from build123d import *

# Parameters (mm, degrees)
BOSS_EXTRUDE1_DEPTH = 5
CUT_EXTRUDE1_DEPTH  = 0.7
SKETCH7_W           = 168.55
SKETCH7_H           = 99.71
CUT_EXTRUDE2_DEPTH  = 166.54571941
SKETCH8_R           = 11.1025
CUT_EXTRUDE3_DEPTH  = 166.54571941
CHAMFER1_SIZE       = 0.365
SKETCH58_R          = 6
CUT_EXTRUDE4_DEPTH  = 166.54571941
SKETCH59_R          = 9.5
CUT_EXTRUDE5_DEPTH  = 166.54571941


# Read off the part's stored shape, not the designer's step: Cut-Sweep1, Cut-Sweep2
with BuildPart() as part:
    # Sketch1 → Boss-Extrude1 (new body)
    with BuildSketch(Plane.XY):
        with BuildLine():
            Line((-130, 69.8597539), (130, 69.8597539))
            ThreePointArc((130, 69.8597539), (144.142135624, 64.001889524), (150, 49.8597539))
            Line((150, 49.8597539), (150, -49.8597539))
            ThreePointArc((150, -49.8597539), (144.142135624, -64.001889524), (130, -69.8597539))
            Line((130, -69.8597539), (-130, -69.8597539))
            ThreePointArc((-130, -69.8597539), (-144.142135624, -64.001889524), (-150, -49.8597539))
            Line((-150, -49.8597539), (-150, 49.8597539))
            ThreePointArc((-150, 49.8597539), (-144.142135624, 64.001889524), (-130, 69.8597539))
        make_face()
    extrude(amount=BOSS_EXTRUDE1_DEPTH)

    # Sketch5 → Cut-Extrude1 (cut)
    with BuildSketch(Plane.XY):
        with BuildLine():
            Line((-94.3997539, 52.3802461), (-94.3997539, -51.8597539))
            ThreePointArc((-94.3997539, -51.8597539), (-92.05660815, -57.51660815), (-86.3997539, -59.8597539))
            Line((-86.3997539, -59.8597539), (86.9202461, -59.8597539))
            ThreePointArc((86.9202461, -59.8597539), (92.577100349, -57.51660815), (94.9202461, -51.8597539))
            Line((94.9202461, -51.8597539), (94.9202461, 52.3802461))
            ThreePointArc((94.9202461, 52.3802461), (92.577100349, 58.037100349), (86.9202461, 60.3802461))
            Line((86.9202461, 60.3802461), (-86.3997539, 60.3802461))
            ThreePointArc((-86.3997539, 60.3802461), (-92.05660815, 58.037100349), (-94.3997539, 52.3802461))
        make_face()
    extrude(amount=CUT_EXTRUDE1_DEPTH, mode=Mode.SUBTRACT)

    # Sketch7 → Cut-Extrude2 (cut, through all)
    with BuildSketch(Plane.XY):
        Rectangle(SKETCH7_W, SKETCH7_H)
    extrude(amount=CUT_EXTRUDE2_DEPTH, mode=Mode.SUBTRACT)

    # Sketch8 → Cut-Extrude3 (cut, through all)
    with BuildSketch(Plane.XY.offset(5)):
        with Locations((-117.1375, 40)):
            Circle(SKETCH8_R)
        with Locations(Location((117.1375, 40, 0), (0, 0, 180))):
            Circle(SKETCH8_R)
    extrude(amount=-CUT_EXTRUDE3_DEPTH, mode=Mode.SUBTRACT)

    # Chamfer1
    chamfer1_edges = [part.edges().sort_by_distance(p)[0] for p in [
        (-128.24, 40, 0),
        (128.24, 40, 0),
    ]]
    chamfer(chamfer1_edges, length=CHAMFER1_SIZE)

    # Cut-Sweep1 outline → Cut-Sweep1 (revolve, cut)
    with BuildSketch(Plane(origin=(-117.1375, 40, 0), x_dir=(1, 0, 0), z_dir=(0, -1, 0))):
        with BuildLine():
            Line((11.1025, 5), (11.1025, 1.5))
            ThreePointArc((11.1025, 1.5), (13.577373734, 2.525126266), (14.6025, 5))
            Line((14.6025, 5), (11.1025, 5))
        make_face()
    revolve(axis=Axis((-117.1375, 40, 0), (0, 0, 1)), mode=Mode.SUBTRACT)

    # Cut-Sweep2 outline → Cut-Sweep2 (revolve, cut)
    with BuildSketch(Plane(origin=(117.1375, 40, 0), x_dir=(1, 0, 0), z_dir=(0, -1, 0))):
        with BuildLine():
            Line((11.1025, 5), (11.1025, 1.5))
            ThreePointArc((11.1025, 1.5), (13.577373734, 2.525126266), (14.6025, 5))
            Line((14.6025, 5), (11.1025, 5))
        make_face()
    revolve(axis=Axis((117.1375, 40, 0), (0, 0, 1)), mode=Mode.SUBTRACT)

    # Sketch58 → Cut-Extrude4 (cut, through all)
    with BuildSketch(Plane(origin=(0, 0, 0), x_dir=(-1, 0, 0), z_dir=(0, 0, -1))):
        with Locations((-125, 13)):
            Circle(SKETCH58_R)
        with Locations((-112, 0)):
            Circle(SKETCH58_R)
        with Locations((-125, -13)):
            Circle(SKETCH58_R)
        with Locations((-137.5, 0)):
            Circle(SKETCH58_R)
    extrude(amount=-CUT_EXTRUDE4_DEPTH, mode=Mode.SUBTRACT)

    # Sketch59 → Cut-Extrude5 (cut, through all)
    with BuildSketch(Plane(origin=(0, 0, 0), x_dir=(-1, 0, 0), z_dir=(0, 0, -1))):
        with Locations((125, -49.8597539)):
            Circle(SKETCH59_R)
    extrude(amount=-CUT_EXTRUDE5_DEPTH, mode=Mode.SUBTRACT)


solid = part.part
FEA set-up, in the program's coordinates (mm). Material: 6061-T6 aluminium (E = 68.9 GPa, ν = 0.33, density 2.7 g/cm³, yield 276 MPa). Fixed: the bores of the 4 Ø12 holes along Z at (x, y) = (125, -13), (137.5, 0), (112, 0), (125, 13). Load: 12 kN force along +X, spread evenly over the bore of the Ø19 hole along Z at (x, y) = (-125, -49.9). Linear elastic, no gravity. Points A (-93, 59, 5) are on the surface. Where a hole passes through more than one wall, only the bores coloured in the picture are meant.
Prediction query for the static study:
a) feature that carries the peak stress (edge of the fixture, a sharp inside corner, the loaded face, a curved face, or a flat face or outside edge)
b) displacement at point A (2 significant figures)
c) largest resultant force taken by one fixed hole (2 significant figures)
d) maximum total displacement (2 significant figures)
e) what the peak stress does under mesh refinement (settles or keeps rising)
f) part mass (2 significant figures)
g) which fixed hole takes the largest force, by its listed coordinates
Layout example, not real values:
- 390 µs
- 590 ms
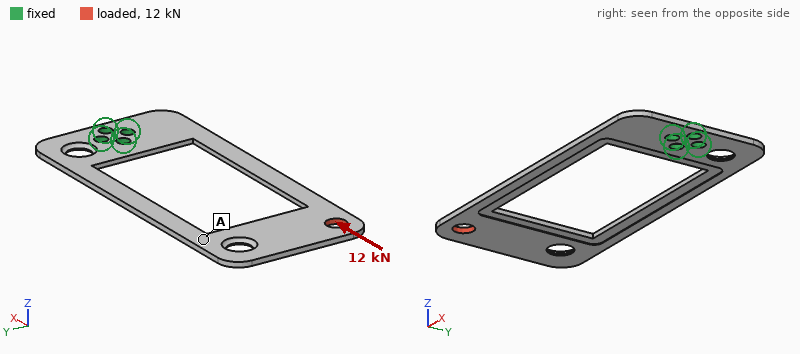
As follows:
- edge of the fixture
- 1.7 mm
- 14 kN
- 2.8 mm
- keeps rising
- 300 g
- (125, -13)
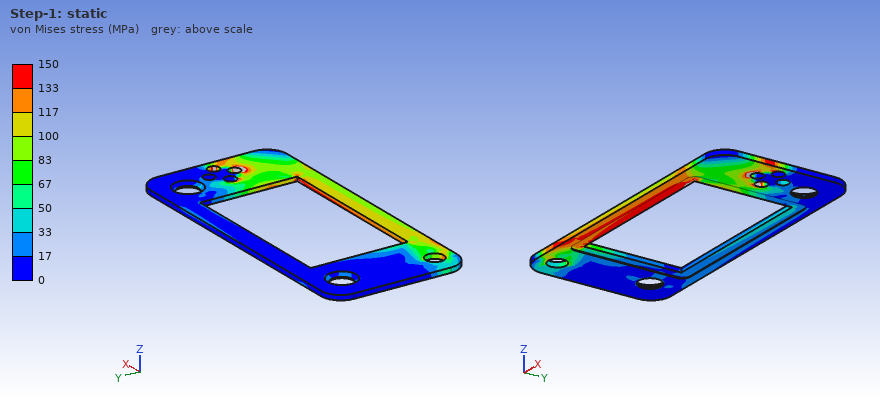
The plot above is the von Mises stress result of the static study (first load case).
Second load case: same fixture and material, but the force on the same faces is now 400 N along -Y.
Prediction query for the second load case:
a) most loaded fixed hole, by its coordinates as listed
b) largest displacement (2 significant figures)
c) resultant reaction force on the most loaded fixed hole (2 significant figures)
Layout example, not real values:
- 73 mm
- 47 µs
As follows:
- (112, 0)
- 0.74 mm
- 1.9 kN
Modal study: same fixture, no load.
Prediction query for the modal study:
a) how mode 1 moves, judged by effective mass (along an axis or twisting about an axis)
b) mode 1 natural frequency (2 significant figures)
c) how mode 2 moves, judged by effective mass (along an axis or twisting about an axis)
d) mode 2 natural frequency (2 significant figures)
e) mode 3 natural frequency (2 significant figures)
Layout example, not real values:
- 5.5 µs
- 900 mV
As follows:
- along Z
- 36 Hz
- twisting about X
- 140 Hz
- 290 Hz
